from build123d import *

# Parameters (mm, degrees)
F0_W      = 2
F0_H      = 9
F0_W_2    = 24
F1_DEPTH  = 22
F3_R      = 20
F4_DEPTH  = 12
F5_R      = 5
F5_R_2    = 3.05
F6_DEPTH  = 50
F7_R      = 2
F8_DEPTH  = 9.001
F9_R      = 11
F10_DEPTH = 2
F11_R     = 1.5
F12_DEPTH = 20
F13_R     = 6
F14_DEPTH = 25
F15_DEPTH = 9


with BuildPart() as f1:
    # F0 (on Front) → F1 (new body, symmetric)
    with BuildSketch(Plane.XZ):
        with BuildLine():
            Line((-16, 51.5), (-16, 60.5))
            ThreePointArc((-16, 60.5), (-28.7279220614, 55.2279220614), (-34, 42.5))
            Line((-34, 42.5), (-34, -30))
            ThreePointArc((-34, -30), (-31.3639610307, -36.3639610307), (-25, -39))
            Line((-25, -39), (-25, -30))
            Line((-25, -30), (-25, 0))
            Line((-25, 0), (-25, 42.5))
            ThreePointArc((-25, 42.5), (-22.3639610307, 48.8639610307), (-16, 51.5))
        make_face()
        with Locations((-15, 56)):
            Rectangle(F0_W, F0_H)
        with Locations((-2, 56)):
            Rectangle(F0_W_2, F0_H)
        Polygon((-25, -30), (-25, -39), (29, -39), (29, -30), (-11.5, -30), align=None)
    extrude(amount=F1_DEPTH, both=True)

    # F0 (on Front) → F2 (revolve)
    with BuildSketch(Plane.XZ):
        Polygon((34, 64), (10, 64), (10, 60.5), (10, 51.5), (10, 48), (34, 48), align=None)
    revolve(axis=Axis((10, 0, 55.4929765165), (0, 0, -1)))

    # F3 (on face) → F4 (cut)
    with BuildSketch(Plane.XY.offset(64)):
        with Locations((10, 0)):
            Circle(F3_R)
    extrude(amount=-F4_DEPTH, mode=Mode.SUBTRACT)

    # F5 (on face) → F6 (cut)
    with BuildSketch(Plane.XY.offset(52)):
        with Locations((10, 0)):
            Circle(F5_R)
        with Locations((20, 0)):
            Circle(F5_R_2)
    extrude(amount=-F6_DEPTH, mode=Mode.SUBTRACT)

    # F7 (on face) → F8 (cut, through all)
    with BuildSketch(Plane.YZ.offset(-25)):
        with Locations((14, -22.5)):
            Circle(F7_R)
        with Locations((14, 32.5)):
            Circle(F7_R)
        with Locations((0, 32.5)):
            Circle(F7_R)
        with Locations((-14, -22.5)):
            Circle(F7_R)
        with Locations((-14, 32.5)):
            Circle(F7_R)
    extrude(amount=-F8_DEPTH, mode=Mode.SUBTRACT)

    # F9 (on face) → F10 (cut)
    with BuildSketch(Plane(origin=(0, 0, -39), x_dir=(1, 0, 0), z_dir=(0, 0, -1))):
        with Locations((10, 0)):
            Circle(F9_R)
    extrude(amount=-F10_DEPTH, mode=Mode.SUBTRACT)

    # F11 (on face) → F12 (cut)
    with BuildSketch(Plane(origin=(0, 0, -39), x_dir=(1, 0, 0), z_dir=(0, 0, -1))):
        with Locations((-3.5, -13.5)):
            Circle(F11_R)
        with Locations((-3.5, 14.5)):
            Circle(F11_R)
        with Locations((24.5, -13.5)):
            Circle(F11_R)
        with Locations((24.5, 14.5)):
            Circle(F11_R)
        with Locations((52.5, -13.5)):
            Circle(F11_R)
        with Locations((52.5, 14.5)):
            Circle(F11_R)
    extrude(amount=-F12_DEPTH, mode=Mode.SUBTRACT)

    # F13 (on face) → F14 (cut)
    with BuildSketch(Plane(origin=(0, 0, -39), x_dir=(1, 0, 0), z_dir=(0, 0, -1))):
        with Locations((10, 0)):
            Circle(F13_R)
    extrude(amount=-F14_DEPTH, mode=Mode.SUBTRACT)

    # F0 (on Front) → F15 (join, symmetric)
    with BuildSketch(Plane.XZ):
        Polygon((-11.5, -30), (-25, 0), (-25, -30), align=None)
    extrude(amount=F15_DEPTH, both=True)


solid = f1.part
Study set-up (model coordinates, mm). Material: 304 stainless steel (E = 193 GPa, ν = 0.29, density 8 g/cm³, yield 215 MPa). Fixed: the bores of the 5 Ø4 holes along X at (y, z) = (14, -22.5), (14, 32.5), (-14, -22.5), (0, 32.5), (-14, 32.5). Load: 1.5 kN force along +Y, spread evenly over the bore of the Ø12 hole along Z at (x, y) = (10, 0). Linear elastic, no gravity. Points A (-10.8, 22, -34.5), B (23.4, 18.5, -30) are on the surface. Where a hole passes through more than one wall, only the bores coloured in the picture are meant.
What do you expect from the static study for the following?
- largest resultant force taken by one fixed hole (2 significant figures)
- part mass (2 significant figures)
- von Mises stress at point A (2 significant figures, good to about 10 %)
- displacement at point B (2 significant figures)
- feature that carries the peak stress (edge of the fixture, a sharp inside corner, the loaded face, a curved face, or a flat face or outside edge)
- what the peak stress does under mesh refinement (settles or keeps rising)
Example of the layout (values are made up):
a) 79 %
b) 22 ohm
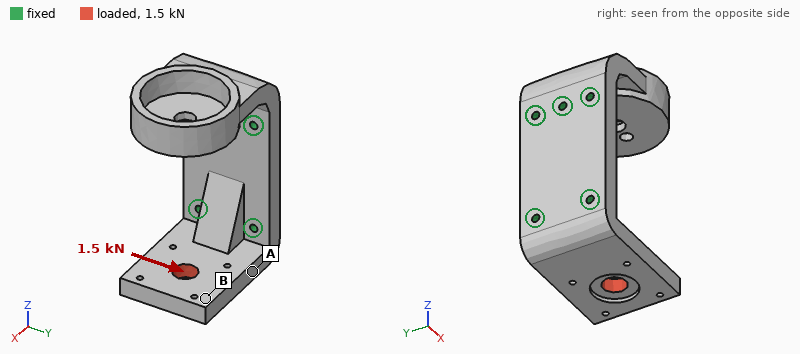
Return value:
a) 2.1 kN
b) 630 g
c) 13 MPa
d) 16 µm
e) edge of the fixture
f) keeps rising
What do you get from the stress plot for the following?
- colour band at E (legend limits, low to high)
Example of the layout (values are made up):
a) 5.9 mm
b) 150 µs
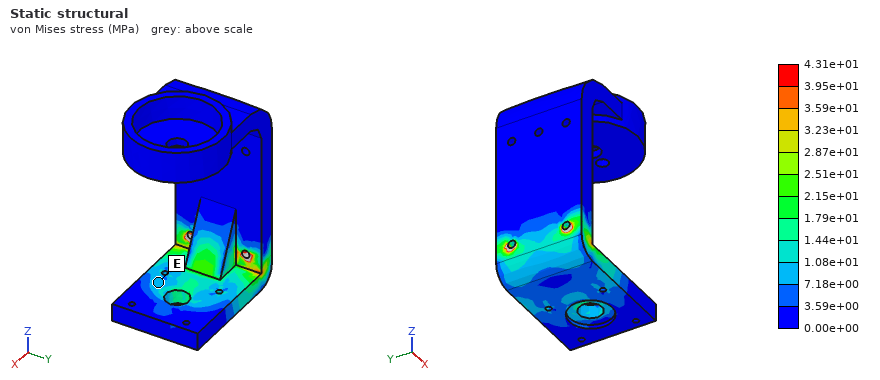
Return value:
a) 7.18e+00 to 1.08e+01 MPa
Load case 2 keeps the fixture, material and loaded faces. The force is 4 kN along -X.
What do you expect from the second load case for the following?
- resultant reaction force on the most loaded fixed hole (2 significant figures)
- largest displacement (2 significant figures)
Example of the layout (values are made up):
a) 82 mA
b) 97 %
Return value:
a) 2.2 kN
b) 16 µm
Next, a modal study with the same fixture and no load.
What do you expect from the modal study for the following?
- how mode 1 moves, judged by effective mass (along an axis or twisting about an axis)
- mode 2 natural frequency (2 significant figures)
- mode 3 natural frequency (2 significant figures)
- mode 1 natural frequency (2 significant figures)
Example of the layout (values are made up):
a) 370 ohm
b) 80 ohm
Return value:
a) along Z
b) 2500 Hz
c) 2600 Hz
d) 1400 Hz
